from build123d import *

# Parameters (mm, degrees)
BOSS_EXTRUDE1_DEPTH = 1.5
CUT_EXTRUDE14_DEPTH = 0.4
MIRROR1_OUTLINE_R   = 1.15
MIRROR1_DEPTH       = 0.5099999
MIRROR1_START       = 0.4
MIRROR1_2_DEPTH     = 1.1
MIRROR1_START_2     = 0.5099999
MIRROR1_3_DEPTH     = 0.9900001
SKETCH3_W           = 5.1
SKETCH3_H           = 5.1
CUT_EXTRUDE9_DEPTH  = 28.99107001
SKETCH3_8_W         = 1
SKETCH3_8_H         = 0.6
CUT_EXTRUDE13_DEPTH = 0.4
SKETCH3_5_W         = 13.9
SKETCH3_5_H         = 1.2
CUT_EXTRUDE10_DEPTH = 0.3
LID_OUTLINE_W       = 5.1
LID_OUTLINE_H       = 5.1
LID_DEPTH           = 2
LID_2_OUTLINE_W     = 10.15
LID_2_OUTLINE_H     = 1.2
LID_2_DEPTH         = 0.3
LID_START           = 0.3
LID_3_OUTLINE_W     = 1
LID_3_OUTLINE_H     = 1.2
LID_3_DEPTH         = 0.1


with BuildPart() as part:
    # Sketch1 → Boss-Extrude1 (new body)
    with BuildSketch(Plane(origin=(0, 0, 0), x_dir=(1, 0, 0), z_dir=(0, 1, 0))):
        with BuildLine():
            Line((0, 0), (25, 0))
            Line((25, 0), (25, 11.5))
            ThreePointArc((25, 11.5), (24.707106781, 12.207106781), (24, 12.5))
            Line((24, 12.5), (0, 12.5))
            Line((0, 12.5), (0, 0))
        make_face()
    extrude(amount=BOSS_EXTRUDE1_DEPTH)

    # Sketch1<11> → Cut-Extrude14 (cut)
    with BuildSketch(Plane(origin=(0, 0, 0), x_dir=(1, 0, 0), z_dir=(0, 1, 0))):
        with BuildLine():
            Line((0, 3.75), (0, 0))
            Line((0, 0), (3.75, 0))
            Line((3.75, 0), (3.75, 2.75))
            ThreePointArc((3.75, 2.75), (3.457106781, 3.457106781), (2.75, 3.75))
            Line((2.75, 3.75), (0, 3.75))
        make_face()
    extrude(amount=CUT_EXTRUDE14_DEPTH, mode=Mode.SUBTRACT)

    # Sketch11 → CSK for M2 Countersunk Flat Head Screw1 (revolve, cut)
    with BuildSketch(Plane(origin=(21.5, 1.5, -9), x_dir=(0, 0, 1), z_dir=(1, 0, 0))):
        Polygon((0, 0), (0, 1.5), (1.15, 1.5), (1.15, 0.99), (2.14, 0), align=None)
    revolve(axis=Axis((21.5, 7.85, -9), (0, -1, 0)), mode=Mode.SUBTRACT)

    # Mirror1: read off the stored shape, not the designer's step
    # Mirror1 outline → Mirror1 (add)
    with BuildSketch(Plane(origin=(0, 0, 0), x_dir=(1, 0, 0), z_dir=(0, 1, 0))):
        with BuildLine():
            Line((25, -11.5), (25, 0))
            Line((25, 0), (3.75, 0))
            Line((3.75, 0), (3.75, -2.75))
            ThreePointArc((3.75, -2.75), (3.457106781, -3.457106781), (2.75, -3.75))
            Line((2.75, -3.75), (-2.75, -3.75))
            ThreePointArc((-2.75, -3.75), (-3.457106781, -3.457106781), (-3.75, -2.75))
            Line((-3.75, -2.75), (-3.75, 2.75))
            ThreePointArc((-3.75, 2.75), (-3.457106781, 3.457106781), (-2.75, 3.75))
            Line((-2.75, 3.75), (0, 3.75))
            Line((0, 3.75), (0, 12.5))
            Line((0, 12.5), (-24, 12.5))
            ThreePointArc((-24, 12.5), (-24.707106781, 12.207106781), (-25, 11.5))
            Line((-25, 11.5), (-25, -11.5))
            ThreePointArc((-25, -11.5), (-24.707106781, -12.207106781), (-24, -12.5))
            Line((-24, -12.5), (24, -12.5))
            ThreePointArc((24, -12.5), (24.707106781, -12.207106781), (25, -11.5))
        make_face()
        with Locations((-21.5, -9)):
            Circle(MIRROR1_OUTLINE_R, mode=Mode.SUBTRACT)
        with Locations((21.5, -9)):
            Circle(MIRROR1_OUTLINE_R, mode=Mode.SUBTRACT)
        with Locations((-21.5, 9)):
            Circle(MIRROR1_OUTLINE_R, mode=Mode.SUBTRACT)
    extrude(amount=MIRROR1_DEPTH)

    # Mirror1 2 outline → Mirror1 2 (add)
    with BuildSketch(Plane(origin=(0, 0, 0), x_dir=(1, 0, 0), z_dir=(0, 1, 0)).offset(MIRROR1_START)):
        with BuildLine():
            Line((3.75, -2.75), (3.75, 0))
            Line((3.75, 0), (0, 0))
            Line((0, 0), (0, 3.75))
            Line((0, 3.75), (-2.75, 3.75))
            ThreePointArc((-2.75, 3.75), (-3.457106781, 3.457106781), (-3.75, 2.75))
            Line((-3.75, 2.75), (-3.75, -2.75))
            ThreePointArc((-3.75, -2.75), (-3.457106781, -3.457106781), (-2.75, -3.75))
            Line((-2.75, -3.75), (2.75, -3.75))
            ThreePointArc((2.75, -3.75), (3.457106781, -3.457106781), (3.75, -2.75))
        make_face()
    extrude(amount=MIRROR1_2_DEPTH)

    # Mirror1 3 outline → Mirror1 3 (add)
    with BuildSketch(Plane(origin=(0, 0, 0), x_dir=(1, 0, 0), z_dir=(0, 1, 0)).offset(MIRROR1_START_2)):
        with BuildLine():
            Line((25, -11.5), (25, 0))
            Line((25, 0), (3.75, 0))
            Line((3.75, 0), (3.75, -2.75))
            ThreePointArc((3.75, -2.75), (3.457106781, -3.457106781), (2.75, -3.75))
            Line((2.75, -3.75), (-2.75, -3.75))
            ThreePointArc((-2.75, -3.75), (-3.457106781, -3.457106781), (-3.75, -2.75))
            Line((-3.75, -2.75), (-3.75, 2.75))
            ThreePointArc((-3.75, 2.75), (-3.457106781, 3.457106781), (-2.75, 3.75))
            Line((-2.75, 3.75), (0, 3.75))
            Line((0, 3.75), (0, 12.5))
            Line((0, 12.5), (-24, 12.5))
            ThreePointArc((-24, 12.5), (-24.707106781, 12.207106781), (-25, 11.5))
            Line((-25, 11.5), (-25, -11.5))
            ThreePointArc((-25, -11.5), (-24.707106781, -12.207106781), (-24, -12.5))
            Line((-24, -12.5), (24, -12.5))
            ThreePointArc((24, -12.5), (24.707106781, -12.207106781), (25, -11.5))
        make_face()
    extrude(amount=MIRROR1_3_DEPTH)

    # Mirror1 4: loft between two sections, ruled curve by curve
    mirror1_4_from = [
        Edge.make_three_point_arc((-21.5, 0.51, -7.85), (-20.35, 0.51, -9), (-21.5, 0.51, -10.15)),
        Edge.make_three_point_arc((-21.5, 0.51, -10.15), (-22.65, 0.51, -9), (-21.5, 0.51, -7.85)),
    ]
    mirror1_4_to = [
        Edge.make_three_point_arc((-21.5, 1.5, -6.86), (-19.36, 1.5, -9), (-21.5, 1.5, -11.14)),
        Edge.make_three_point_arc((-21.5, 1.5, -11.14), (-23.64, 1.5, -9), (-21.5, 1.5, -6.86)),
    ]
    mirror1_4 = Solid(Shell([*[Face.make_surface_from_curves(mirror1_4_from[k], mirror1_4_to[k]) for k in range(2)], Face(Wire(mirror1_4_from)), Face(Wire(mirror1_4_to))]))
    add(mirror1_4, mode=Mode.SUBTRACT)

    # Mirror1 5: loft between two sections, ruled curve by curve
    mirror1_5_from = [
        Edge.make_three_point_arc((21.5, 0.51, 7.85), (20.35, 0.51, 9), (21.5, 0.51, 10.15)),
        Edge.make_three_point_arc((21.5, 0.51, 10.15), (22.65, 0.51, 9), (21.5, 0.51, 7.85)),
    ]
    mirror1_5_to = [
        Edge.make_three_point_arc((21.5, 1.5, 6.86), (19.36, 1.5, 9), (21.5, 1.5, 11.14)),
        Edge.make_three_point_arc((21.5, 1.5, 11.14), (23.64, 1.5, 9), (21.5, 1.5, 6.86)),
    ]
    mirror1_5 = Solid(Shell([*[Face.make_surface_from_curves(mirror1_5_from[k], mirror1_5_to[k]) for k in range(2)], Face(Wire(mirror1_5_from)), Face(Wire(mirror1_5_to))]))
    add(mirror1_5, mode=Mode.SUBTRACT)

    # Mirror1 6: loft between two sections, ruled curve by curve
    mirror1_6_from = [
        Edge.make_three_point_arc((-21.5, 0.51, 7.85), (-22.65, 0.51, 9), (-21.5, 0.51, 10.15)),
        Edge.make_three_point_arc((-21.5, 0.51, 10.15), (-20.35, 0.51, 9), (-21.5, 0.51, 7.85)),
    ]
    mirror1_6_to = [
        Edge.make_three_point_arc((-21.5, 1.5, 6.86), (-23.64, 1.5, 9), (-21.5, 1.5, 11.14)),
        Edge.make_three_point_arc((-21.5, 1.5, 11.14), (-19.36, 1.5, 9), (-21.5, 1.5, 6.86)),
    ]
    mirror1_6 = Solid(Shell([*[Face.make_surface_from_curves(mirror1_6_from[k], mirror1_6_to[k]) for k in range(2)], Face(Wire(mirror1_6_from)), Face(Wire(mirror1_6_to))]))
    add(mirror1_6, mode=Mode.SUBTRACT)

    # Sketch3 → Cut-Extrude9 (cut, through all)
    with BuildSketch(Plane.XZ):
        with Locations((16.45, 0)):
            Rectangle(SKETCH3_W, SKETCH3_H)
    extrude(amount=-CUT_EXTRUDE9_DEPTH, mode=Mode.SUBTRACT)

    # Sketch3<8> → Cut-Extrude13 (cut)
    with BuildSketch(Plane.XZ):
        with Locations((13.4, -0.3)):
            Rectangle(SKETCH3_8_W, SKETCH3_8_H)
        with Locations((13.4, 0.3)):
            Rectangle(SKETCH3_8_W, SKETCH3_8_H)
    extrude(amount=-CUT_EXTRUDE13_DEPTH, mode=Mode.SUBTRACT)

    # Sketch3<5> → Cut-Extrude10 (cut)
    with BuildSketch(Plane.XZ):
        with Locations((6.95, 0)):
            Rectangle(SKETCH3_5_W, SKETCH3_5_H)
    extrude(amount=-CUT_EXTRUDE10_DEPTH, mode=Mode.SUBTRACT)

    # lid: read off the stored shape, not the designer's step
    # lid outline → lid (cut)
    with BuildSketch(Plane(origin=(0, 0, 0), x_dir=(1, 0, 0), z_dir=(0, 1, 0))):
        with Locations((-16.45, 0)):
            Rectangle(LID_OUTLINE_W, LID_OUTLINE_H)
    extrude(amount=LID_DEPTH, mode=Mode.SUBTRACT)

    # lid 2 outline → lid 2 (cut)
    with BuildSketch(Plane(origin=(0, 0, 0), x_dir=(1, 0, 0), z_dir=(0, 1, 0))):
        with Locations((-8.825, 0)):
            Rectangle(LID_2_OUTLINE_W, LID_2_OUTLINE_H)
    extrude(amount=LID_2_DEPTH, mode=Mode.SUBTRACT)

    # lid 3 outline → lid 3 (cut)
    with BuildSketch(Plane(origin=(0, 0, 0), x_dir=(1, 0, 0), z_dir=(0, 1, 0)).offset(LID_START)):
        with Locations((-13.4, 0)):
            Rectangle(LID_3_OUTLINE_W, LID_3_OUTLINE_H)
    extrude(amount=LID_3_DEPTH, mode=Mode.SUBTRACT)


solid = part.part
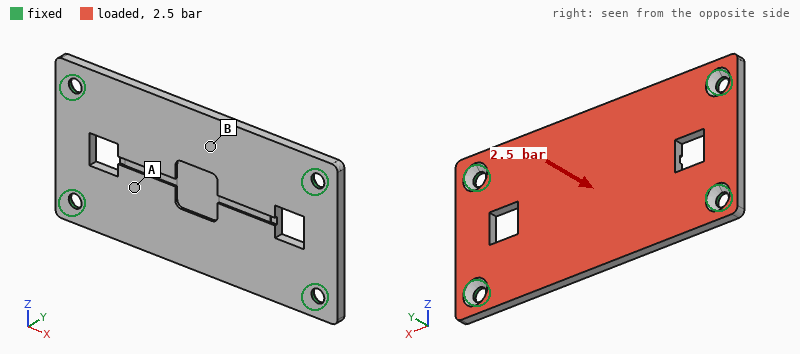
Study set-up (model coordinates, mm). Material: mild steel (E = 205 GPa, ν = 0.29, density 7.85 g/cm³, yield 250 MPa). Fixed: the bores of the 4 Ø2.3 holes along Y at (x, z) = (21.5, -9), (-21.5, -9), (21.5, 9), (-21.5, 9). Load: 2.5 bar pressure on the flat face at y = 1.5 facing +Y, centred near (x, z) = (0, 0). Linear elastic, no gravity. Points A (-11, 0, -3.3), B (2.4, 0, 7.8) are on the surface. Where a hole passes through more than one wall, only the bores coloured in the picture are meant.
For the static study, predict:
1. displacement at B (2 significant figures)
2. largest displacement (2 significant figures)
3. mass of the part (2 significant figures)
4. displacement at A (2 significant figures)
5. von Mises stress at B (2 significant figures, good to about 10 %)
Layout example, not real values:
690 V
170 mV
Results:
56 µm
58 µm
14 g
35 µm
58 MPa
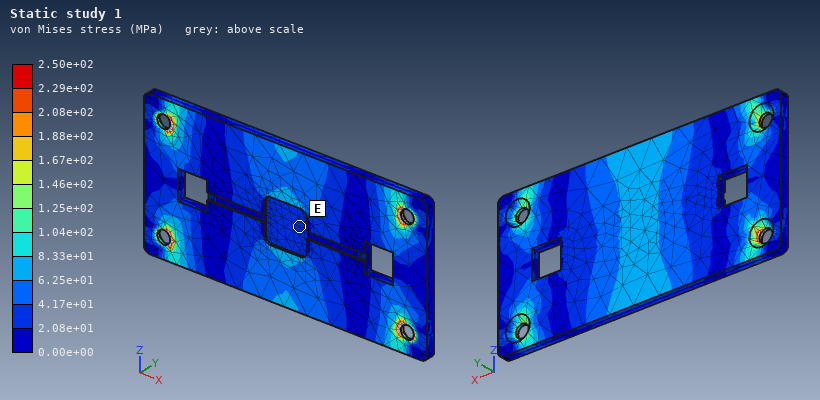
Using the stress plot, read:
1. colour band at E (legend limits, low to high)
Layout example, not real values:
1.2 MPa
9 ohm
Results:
2.08e+01 to 4.17e+01 MPa
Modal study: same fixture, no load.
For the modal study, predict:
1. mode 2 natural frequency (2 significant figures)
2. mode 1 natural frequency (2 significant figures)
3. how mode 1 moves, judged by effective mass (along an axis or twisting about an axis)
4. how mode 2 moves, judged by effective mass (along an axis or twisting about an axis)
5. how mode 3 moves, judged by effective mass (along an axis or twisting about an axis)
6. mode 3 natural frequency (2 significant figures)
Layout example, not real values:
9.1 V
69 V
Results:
5800 Hz
3500 Hz
along Y
twisting about X
twisting about Z
9700 Hz
